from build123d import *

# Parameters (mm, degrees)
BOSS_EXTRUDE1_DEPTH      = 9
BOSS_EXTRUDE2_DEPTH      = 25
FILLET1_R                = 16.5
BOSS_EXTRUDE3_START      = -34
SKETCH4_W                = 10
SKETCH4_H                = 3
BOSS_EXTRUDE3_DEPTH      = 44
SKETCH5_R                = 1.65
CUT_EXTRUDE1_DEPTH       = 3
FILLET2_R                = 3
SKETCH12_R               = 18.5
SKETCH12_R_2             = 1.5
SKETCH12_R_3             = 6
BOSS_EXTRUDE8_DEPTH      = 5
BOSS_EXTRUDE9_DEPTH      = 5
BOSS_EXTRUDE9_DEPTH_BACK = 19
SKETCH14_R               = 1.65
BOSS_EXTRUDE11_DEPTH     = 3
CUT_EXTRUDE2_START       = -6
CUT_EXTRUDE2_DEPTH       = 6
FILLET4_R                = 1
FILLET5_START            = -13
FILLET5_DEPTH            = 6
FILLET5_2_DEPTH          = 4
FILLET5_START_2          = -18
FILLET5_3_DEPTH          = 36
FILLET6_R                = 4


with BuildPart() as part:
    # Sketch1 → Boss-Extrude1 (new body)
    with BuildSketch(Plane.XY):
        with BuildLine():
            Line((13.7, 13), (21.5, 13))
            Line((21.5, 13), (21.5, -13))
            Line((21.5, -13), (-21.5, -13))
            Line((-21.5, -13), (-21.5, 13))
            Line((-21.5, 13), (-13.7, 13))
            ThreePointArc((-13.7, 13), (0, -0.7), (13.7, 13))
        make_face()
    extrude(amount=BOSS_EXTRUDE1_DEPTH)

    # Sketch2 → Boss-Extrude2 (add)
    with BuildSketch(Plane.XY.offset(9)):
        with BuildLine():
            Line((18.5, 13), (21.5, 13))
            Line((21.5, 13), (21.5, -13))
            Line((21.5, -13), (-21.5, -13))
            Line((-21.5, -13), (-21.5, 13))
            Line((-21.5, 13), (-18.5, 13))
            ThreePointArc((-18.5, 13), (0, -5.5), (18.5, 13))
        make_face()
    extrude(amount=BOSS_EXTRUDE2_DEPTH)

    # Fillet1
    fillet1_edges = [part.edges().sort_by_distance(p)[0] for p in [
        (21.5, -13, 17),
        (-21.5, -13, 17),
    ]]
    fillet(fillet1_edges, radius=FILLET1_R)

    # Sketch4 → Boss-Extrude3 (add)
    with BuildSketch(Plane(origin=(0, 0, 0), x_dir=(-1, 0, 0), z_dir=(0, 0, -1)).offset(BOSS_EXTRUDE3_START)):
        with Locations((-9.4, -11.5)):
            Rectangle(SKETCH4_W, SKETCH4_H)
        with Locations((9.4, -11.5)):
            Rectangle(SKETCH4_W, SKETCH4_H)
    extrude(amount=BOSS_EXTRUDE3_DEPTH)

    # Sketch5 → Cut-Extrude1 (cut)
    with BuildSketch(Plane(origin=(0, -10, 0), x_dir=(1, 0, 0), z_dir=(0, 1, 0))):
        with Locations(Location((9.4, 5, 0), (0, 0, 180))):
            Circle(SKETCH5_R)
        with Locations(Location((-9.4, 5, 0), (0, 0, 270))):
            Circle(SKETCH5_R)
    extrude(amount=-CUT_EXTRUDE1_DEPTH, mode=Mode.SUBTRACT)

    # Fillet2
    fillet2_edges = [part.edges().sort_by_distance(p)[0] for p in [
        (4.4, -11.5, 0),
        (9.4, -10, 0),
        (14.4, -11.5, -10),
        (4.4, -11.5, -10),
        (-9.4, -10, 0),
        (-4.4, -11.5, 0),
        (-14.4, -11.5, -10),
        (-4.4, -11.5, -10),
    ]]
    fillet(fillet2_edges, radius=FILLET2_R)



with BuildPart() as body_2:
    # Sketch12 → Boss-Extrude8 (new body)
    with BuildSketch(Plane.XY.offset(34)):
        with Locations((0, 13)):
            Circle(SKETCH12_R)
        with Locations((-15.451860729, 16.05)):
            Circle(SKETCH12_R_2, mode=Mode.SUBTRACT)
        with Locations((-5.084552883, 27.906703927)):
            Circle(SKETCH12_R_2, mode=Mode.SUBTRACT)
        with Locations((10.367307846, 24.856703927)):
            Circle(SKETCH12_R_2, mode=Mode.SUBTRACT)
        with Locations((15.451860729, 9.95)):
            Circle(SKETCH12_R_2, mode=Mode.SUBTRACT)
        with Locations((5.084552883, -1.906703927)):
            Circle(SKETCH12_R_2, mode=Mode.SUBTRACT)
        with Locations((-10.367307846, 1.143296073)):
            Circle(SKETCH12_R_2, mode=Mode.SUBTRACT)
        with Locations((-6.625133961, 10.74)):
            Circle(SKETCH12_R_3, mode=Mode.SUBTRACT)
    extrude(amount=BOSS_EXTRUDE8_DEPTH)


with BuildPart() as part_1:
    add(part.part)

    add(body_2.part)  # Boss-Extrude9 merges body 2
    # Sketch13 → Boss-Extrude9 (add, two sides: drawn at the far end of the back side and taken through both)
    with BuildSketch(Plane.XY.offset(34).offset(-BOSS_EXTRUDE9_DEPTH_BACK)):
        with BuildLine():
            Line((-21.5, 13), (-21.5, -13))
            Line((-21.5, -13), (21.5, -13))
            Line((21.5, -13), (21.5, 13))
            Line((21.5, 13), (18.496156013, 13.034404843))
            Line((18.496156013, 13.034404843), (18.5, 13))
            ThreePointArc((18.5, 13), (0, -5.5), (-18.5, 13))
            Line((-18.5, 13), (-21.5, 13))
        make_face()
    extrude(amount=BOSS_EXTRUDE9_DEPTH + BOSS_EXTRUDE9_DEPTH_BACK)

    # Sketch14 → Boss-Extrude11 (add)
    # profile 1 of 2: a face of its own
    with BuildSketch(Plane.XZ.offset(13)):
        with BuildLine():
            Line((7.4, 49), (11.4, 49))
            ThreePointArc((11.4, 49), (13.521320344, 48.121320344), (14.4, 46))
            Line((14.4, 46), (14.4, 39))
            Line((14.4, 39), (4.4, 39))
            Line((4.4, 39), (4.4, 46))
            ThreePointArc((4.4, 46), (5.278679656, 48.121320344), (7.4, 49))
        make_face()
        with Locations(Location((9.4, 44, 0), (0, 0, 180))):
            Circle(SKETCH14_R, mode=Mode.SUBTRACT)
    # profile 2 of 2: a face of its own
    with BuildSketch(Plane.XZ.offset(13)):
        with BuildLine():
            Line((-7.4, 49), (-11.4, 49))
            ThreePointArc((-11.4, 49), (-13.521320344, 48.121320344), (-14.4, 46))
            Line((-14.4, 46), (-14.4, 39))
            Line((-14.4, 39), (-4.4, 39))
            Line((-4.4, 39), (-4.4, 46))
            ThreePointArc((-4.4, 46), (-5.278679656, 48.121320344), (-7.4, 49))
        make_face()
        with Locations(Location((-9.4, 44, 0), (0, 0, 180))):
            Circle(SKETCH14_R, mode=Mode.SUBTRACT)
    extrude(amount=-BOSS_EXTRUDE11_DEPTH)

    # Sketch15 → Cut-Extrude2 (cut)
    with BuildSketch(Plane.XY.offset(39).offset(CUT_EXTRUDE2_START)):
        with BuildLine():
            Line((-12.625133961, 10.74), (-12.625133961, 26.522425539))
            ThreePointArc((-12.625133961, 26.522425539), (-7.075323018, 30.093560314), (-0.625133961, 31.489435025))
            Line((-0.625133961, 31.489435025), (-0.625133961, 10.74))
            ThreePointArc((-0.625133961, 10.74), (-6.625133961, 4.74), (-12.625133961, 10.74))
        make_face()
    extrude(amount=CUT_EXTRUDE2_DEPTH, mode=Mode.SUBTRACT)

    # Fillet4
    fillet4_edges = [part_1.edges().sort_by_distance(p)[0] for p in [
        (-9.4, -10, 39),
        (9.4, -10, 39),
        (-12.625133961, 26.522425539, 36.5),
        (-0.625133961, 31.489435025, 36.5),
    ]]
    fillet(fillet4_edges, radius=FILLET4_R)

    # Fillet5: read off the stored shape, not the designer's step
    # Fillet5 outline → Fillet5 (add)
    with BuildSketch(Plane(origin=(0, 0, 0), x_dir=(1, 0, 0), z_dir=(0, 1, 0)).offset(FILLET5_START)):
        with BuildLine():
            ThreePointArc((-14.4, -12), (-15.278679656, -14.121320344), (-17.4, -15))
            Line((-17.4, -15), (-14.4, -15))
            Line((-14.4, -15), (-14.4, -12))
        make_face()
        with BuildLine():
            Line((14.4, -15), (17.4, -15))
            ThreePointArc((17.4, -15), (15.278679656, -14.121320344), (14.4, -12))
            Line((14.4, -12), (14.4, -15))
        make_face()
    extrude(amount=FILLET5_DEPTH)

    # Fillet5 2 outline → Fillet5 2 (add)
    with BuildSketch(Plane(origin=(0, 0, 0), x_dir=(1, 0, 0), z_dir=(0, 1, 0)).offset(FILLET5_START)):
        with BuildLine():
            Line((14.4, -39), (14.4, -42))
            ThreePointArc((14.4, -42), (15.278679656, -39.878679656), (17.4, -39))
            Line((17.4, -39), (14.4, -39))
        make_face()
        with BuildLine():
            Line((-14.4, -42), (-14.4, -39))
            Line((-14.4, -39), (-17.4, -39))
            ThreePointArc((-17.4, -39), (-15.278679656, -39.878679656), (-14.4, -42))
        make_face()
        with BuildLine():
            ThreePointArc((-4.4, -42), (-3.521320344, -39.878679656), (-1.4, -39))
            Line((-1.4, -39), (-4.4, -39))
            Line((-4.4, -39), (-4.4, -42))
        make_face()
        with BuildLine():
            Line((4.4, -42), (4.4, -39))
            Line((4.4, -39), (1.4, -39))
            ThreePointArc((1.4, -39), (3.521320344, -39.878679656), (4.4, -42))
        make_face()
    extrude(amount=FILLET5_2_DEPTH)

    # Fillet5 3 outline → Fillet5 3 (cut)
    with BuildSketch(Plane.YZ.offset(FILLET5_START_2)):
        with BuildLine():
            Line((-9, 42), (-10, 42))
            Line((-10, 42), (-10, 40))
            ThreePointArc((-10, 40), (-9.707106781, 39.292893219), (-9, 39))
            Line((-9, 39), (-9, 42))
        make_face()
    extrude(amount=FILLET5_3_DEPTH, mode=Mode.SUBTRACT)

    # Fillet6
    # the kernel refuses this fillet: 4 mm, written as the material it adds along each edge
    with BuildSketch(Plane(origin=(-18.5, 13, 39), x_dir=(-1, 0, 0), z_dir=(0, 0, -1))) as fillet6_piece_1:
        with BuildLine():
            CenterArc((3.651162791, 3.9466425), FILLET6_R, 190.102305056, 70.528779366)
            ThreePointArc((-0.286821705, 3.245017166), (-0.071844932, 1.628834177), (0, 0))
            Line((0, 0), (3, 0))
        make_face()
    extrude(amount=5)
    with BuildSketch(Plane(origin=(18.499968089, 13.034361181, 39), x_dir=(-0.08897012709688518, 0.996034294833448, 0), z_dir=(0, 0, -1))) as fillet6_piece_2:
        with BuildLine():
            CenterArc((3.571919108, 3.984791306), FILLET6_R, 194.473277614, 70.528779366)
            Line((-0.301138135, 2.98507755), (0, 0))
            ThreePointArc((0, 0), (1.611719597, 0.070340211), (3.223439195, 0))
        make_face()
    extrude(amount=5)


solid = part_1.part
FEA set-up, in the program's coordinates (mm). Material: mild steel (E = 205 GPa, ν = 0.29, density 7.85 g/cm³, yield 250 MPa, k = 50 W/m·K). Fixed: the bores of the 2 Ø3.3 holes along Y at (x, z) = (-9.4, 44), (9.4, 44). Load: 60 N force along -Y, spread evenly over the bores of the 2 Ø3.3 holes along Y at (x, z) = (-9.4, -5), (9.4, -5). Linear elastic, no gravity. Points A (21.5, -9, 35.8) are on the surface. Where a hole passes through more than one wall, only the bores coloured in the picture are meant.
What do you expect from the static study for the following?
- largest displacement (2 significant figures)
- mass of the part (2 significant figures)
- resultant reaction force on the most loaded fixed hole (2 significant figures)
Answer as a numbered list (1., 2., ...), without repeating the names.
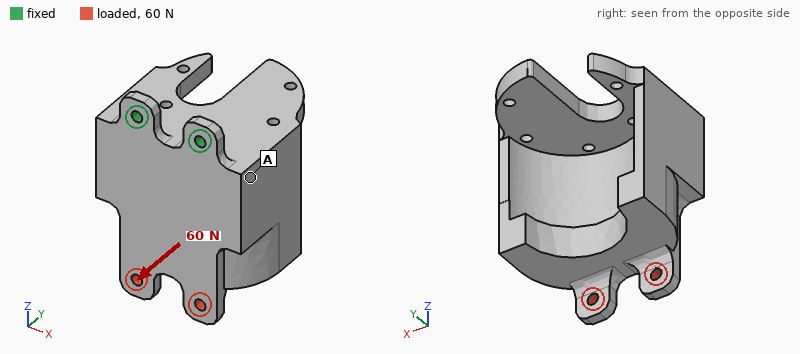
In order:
1. 76 µm
2. 220 g
3. 31 N
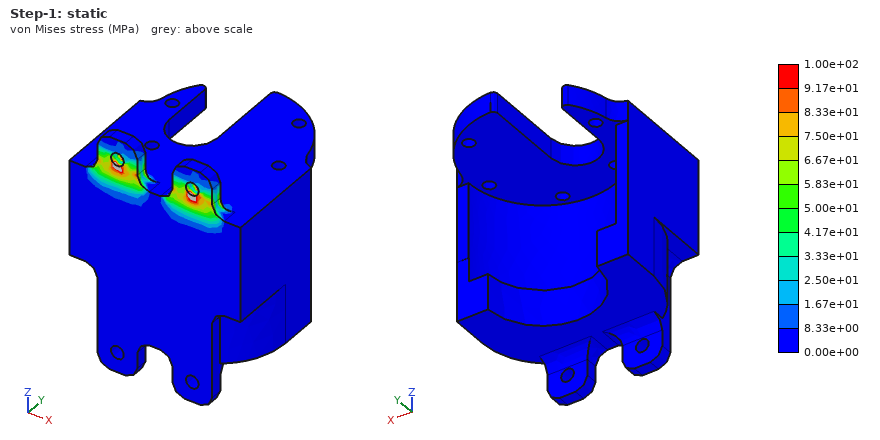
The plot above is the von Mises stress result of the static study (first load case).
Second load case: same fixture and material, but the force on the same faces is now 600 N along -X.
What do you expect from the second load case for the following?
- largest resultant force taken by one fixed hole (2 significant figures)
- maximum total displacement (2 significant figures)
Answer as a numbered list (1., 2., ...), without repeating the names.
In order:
1. 1.4 kN
2. 19 µm
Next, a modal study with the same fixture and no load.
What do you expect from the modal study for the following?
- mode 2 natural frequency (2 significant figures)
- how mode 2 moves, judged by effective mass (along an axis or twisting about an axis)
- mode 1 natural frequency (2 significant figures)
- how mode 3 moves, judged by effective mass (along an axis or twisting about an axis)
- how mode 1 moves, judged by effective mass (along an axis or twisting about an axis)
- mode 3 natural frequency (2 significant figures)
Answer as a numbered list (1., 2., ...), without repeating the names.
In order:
1. 2900 Hz
2. along X
3. 550 Hz
4. along X
5. along Y
6. 3900 Hz
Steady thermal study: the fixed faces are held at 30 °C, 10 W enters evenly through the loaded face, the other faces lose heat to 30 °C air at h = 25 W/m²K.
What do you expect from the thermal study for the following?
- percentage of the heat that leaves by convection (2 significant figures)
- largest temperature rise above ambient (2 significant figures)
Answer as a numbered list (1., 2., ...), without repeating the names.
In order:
1. 42 %
2. 50 K
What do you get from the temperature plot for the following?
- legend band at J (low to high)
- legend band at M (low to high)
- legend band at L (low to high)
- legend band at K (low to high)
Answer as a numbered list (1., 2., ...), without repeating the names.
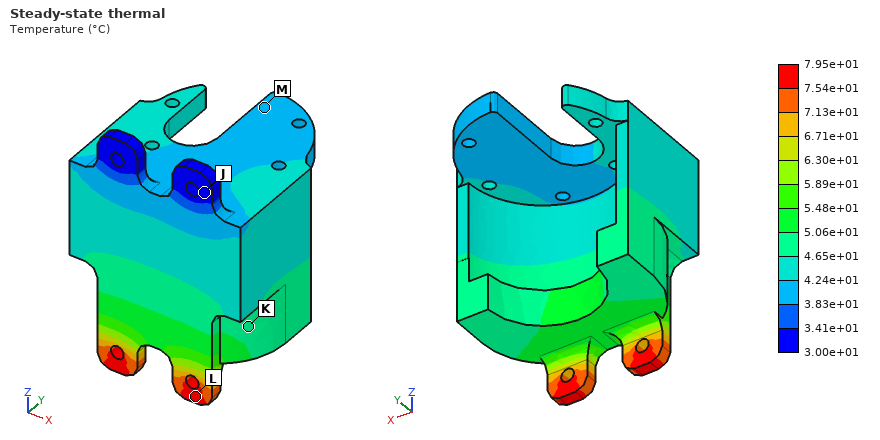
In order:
1. 3.00e+01 to 3.41e+01 °C
2. 3.83e+01 to 4.24e+01 °C
3. 7.54e+01 to 7.95e+01 °C
4. 4.65e+01 to 5.06e+01 °C
